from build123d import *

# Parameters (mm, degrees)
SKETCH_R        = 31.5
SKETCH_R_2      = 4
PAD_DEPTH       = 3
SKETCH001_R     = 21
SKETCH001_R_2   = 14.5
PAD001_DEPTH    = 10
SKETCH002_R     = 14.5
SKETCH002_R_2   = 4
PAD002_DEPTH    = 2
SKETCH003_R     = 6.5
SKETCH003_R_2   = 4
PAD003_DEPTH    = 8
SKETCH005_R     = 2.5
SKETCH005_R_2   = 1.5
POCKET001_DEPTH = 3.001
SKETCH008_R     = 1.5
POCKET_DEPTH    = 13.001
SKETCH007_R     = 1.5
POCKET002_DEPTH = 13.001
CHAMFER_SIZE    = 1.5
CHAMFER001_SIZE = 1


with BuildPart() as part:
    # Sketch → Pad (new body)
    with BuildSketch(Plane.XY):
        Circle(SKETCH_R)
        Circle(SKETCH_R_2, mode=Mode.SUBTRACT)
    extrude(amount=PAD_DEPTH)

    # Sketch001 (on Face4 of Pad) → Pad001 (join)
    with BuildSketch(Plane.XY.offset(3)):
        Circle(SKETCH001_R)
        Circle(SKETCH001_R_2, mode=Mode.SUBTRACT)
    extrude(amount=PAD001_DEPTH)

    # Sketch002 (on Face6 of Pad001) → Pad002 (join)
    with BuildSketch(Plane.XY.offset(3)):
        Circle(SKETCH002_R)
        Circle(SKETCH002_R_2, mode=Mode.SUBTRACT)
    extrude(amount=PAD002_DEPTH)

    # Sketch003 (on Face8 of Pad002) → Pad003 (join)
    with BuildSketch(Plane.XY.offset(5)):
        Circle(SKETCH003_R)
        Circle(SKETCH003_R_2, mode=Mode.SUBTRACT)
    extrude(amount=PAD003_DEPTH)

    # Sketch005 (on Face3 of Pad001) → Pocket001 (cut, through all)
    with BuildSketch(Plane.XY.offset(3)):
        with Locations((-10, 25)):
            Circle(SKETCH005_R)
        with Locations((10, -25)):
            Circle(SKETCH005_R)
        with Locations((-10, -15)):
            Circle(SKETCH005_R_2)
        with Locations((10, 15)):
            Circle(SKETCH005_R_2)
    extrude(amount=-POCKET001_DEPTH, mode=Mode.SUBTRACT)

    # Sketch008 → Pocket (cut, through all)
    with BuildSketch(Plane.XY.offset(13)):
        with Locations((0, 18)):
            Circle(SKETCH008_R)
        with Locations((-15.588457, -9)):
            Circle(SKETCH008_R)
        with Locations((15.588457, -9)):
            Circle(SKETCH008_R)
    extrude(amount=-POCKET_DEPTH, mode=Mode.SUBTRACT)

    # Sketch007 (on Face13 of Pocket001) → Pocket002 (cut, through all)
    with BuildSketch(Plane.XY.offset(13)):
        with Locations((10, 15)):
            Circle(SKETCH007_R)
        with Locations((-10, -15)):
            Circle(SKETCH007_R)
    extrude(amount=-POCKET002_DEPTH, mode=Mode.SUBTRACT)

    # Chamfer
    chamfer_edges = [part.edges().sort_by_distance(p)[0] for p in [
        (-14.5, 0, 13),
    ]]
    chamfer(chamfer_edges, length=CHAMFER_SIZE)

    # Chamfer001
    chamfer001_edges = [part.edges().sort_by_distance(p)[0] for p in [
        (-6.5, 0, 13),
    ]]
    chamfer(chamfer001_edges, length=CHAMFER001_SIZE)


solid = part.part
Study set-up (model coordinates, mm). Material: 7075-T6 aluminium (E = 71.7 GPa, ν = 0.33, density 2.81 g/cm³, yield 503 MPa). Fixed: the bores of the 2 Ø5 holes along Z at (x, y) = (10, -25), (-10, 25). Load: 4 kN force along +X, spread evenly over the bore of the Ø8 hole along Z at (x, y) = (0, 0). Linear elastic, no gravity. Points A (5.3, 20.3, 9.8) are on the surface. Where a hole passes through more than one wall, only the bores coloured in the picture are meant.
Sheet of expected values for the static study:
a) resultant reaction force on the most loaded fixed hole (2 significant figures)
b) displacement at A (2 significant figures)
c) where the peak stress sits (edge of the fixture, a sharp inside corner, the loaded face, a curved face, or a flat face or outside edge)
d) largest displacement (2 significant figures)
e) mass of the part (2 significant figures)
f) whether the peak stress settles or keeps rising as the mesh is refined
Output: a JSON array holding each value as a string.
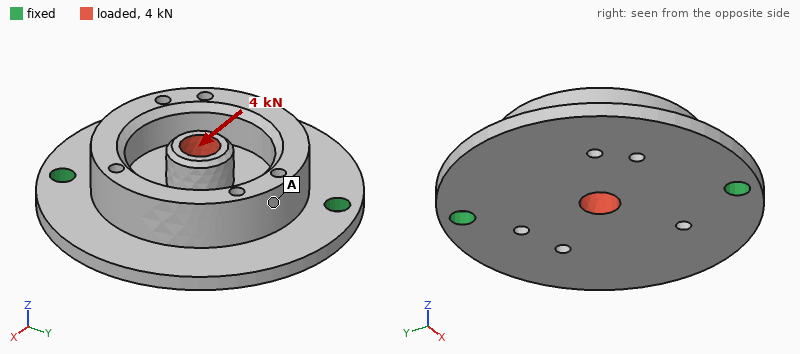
["2.0 kN", "0.12 mm", "edge of the fixture", "0.26 mm", "50 g", "keeps rising"]
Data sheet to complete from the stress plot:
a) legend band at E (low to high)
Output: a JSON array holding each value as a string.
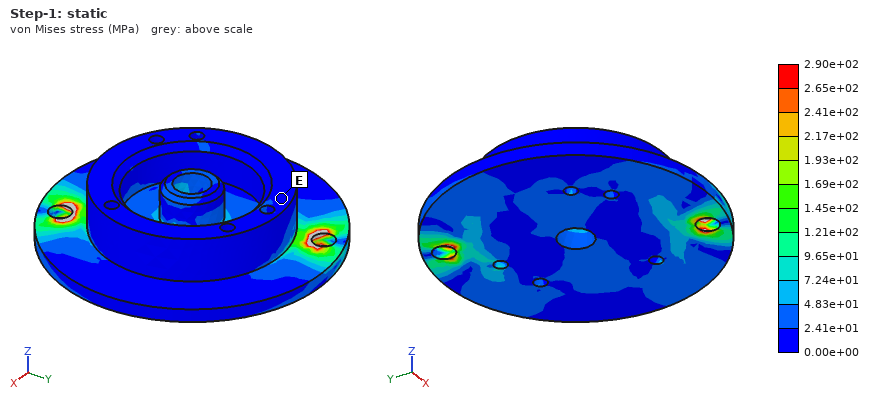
["0.00e+00 to 2.41e+01 MPa"]
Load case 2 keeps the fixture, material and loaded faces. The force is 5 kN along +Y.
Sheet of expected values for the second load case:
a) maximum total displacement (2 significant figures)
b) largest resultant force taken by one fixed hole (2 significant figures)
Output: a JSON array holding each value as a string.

["0.13 mm", "2.6 kN"]
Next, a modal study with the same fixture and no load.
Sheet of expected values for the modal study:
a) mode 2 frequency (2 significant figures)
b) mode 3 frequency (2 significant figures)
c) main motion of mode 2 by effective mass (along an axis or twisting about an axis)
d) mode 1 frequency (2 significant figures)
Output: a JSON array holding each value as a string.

["5300 Hz", "11 kHz", "along Z", "2300 Hz"]
